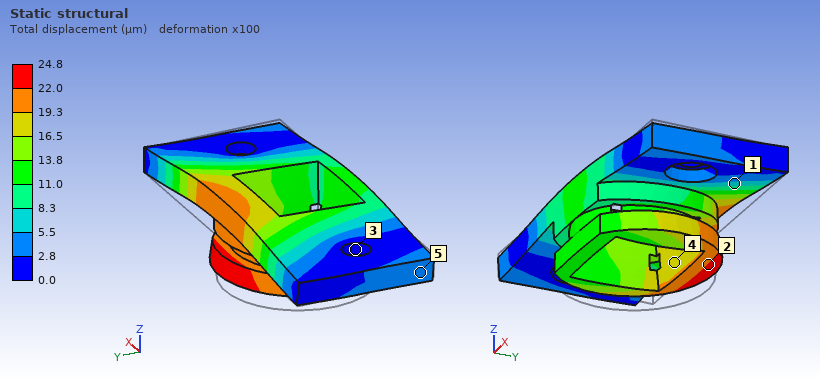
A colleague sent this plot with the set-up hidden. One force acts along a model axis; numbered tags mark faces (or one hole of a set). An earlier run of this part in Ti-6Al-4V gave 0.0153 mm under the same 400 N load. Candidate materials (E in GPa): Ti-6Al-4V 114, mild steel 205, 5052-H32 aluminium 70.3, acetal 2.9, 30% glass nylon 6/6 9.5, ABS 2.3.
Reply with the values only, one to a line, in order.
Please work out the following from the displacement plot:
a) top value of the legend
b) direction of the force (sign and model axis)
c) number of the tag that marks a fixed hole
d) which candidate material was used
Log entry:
24.8 µm
+Z
3
5052-H32 aluminium
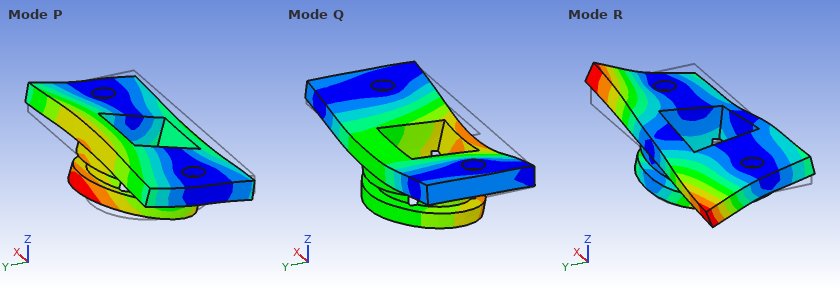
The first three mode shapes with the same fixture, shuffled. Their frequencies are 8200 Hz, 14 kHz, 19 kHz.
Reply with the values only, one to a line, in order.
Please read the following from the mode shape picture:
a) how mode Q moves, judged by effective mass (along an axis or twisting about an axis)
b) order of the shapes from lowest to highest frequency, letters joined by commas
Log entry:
along Z
P, Q, R
